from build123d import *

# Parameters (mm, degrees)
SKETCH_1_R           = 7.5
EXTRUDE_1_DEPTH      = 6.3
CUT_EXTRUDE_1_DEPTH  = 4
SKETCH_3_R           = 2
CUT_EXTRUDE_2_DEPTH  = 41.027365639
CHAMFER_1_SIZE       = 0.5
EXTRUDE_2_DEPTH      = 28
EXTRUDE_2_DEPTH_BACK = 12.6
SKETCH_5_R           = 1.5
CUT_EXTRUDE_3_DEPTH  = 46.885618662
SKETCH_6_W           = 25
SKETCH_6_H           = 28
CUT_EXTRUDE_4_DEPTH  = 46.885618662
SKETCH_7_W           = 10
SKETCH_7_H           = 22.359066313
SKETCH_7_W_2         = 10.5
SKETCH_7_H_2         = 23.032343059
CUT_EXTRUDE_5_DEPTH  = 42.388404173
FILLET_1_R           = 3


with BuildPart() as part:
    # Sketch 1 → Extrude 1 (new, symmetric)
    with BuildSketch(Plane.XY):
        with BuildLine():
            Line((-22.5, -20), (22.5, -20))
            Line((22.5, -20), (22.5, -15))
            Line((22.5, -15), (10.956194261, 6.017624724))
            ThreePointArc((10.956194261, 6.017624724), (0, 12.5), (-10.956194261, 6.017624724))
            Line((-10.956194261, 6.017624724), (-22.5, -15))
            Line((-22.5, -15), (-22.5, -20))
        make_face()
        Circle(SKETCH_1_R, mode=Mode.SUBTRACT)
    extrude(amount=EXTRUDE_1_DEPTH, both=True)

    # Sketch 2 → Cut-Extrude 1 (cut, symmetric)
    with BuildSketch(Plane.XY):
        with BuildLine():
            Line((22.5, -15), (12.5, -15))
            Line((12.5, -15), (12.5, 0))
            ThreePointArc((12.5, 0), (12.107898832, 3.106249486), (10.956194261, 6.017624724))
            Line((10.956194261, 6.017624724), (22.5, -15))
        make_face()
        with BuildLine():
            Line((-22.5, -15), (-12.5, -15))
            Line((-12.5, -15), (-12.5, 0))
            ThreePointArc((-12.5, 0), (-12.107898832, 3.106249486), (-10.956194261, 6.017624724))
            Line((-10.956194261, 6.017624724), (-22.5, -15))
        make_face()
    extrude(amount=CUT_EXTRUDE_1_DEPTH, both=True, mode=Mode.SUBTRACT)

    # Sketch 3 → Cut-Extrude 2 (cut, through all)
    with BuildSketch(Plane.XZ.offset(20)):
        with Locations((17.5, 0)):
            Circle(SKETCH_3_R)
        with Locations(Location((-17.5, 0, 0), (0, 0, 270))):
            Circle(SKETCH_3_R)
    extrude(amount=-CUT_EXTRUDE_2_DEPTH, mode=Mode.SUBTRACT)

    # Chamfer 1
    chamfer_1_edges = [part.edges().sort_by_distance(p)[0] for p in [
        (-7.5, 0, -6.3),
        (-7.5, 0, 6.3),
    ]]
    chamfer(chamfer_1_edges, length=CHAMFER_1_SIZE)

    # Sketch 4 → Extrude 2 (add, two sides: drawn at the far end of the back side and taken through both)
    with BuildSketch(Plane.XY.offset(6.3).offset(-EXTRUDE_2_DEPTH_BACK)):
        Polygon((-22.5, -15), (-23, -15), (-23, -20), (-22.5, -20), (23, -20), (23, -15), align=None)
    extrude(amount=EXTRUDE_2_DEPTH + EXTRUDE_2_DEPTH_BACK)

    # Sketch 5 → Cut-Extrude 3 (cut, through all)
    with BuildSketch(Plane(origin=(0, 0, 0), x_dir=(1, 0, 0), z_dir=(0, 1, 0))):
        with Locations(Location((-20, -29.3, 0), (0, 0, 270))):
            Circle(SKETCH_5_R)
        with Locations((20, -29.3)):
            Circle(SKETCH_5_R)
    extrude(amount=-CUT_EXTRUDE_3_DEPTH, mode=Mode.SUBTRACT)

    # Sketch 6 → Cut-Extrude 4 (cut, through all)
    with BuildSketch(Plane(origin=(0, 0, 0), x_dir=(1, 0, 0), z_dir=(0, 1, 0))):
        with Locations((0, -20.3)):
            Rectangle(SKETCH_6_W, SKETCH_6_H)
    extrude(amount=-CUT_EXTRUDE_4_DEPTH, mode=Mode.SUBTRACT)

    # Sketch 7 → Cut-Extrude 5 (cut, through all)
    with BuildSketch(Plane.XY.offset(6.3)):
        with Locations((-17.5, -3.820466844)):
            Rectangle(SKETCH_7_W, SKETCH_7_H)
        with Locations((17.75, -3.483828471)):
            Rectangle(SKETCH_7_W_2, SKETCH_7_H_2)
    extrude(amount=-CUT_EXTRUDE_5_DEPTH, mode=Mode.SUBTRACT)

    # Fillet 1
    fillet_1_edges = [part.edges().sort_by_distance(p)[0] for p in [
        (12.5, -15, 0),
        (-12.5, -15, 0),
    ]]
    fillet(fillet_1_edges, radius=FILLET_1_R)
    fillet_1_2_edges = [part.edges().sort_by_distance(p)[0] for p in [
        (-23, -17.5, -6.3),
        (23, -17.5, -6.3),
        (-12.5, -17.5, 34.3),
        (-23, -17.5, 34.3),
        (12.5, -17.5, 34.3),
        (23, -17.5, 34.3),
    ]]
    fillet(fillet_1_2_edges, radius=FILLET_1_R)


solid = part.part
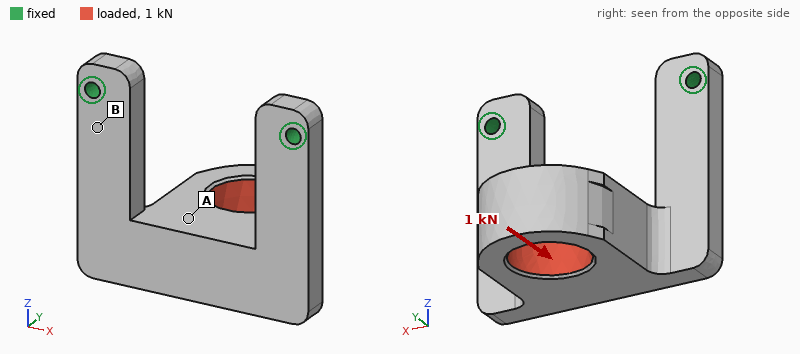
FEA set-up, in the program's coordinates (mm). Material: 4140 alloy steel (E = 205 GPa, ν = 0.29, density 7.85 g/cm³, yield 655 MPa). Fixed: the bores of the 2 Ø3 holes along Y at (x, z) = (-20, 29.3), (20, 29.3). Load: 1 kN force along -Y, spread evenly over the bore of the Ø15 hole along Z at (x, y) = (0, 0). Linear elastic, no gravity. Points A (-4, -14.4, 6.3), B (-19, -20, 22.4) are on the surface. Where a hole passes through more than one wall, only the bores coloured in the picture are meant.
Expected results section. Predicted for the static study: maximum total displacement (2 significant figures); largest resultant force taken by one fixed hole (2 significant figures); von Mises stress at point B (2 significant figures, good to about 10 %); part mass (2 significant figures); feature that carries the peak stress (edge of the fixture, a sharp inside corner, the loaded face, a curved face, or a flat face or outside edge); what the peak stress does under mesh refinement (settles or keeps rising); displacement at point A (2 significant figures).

0.39 mm
500 N
260 MPa
89 g
edge of the fixture
keeps rising
0.14 mm
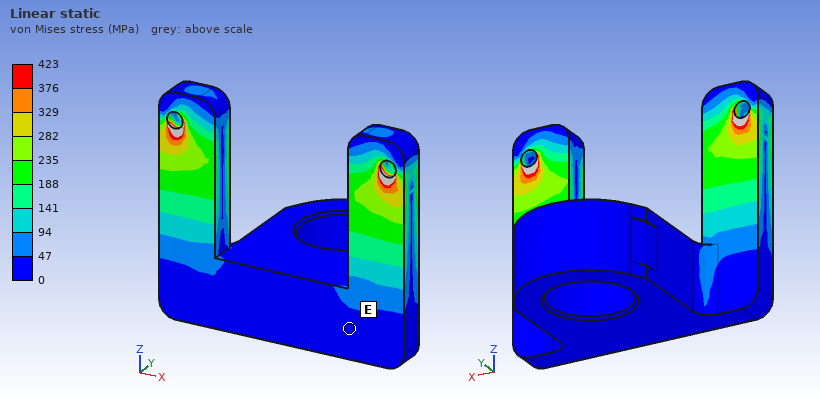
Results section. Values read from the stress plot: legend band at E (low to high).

0 to 47 MPa
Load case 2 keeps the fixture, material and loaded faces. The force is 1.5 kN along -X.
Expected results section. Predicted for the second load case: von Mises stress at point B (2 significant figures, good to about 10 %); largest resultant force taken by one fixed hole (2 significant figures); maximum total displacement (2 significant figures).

130 MPa
1.2 kN
0.13 mm
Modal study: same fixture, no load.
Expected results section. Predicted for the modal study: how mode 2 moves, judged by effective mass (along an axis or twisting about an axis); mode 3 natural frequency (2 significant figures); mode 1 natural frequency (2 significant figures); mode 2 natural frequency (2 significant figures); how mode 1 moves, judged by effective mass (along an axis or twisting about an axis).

along X
4200 Hz
1100 Hz
2900 Hz
along Y
